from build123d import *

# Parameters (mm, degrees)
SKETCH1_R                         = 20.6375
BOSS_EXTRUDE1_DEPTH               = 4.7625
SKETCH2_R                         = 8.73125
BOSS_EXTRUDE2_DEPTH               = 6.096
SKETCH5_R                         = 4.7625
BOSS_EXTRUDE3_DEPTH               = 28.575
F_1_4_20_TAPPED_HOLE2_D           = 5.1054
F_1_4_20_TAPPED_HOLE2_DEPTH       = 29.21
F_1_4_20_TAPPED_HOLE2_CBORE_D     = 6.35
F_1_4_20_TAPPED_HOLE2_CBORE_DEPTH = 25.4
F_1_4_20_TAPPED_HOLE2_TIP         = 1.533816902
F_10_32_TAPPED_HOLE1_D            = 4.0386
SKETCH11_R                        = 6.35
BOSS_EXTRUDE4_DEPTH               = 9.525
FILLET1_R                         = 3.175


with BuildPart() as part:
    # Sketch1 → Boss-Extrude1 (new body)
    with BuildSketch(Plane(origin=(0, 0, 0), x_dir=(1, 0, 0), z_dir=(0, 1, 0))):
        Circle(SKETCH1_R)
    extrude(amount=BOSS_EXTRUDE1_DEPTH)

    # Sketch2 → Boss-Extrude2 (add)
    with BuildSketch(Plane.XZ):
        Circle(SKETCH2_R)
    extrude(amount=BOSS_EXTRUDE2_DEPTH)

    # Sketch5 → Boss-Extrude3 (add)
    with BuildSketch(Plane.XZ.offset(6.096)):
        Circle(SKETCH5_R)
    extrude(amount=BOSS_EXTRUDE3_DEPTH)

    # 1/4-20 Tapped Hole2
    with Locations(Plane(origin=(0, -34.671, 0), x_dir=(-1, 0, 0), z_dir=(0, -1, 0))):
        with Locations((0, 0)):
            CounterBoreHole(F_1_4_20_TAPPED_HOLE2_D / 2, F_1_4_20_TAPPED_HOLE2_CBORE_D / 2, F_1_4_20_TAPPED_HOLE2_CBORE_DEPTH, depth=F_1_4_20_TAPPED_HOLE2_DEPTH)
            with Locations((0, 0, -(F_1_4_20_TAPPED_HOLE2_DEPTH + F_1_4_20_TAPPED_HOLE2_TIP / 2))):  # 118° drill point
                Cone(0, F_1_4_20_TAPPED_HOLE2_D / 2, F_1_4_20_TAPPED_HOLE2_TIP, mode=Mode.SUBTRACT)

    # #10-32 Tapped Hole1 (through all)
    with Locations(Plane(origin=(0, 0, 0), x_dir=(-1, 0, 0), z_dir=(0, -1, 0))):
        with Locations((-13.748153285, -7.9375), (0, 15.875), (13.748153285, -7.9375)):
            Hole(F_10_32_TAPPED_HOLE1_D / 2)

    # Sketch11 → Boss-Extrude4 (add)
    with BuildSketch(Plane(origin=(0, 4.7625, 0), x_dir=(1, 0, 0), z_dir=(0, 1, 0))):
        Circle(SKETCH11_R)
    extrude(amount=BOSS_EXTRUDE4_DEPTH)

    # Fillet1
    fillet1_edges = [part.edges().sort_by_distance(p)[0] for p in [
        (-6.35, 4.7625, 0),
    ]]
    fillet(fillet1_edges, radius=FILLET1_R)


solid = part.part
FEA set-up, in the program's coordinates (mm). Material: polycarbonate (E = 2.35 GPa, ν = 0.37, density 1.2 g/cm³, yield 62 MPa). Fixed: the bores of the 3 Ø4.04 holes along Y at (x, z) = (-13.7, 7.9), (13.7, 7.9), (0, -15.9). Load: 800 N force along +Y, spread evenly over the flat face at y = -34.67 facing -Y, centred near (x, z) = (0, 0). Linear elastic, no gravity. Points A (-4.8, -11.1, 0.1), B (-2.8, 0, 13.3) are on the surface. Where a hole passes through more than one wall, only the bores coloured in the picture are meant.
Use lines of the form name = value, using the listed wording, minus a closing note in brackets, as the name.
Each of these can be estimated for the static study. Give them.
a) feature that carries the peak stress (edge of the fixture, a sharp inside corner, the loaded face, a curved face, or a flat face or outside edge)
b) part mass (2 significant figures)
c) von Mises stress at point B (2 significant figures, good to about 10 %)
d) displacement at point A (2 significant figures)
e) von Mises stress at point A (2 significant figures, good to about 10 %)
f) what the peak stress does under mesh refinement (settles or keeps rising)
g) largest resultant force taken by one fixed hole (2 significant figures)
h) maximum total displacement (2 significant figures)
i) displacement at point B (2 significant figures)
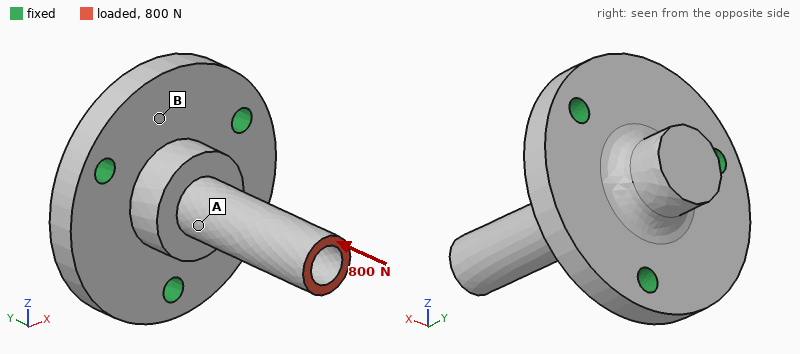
feature that carries the peak stress = edge of the fixture
part mass = 12 g
von Mises stress at point B = 4.4 MPa
displacement at point A = 0.14 mm
von Mises stress at point A = 19 MPa
what the peak stress does under mesh refinement = keeps rising
largest resultant force taken by one fixed hole = 270 N
maximum total displacement = 0.34 mm
displacement at point B = 0.058 mm
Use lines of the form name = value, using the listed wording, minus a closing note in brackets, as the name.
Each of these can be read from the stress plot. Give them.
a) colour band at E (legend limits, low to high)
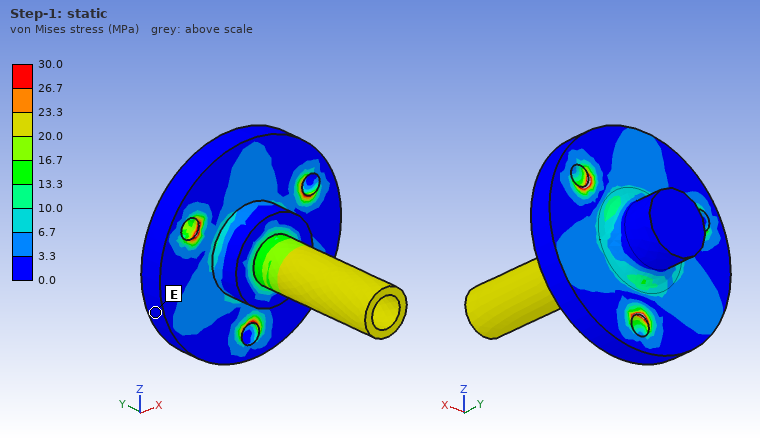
colour band at E = 0.0 to 3.3 MPa
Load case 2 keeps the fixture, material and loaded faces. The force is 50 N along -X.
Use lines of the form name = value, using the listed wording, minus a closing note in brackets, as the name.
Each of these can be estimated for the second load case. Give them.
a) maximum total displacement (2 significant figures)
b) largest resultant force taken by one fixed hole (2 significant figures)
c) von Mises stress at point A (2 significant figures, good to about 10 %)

maximum total displacement = 0.77 mm
largest resultant force taken by one fixed hole = 73 N
von Mises stress at point A = 17 MPa
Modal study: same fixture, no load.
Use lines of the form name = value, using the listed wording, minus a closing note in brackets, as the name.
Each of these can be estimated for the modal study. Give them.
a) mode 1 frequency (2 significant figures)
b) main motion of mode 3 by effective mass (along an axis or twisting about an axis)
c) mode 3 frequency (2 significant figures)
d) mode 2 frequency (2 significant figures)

mode 1 frequency = 2100 Hz
main motion of mode 3 by effective mass = along Y
mode 3 frequency = 5200 Hz
mode 2 frequency = 2100 Hz
